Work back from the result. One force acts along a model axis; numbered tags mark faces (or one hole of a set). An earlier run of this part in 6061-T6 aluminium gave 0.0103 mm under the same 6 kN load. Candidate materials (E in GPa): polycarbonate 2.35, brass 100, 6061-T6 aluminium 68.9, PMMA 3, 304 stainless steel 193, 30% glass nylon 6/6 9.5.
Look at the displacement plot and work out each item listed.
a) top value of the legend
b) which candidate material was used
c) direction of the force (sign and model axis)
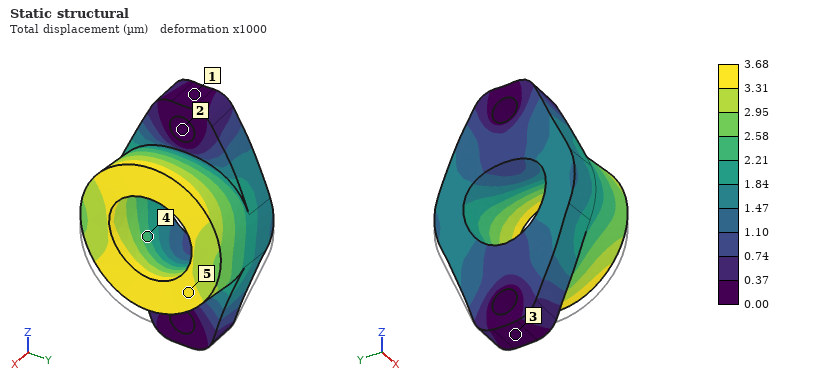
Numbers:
3.68 µm
304 stainless steel
+Z
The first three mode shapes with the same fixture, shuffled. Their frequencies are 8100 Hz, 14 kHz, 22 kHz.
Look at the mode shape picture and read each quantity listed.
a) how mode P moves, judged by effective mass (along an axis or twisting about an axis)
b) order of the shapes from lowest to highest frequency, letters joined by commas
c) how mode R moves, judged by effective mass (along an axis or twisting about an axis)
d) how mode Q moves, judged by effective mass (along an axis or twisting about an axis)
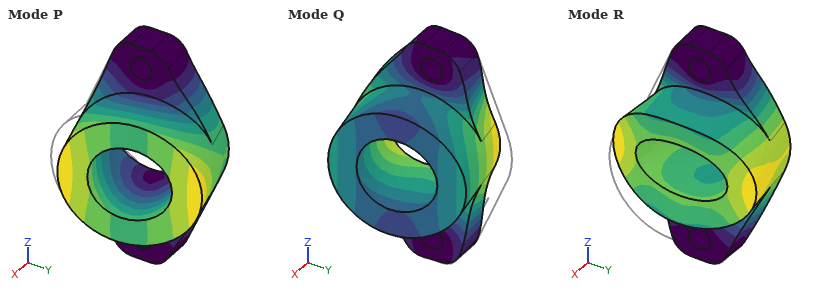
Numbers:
along Y
P, R, Q
along X
along Y
